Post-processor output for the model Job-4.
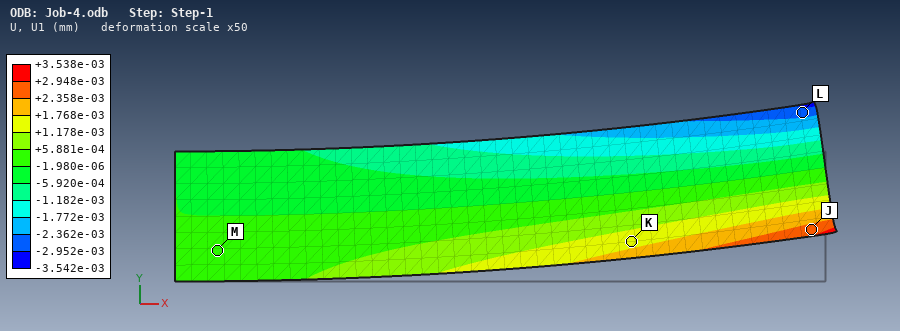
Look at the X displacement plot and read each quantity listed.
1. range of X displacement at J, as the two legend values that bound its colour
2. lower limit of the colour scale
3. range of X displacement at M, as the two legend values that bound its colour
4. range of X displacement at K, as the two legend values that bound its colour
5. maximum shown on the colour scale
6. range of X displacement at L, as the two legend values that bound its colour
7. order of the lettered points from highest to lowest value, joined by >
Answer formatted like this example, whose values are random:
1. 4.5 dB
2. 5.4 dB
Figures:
1. +2.358e-03 to +2.948e-03 mm
2. -3.542e-03 mm
3. -1.980e-06 to +5.881e-04 mm
4. +1.178e-03 to +1.768e-03 mm
5. +3.538e-03 mm
6. -2.952e-03 to -2.362e-03 mm
7. J > K > M > L
